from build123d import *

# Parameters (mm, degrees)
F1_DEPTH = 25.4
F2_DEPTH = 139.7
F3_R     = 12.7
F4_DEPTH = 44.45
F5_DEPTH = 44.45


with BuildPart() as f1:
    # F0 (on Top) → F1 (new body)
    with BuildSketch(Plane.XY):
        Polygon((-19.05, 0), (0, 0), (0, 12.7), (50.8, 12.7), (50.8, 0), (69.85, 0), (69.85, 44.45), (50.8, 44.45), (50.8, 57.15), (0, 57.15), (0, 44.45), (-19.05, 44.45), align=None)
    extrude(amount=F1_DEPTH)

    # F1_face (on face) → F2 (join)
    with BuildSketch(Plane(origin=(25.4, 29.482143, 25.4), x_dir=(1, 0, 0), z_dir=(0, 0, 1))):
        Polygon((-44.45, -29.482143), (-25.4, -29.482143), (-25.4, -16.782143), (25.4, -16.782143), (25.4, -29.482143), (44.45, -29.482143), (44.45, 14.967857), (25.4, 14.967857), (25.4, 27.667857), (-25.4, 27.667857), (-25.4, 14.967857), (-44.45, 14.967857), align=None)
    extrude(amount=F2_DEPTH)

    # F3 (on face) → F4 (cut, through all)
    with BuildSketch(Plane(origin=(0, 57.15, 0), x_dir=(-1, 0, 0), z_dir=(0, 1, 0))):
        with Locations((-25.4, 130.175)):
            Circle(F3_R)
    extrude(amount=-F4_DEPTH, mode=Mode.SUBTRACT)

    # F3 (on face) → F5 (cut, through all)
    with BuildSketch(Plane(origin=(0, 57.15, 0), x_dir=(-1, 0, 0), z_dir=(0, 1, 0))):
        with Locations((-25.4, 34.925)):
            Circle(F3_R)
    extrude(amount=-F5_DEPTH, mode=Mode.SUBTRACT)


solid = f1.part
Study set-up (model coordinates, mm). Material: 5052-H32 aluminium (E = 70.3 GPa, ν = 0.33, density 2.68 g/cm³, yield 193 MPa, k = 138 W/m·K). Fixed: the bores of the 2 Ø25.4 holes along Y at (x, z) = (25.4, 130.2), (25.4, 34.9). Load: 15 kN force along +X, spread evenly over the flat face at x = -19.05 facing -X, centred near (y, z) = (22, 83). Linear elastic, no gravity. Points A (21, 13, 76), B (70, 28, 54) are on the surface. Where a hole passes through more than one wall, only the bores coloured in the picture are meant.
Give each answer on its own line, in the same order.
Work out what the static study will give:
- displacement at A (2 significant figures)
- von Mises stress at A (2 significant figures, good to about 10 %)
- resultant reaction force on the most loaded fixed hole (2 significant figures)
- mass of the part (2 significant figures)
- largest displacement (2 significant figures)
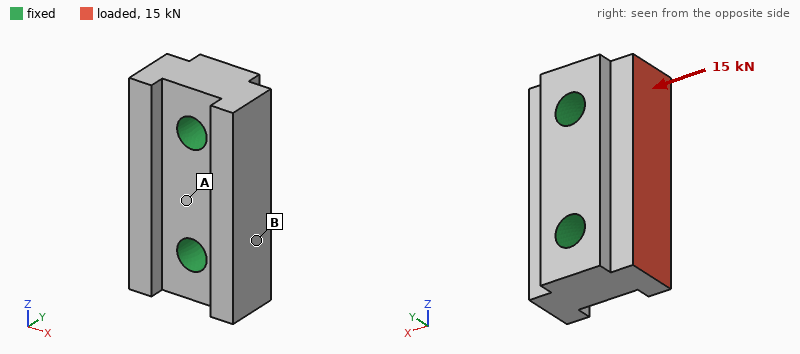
1.9 µm
2.6 MPa
7.6 kN
1.6 kg
6.7 µm
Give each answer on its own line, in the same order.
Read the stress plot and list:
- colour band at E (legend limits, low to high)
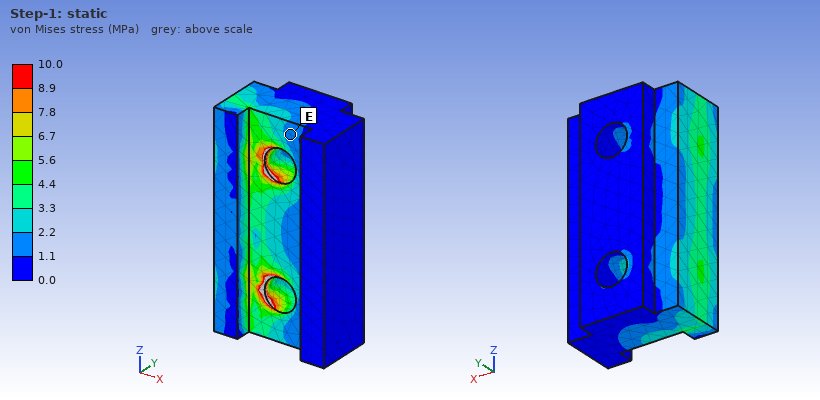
1.1 to 2.2 MPa
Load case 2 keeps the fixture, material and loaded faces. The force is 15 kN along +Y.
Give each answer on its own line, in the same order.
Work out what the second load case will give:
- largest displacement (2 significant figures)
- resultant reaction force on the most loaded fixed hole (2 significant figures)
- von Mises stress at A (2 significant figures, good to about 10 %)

17 µm
7.5 kN
5.2 MPa
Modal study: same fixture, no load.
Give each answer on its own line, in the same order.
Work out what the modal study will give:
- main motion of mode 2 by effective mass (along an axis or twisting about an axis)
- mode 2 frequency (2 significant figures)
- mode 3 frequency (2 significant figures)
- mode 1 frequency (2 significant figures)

along Y
11 kHz
12 kHz
9800 Hz
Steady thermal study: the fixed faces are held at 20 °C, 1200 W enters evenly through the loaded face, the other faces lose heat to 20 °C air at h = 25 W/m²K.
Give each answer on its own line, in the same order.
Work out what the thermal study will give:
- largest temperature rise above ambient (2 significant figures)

68 K
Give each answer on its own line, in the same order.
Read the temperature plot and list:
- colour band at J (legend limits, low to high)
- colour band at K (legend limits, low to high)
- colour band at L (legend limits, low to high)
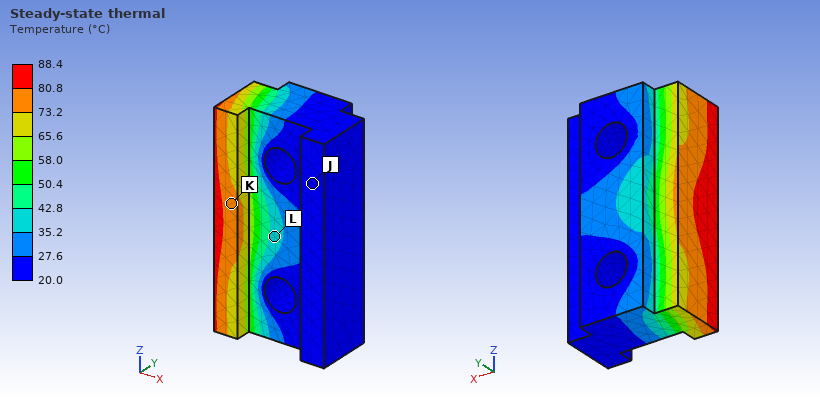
20.0 to 27.6 °C
73.2 to 80.8 °C
35.2 to 42.8 °C
